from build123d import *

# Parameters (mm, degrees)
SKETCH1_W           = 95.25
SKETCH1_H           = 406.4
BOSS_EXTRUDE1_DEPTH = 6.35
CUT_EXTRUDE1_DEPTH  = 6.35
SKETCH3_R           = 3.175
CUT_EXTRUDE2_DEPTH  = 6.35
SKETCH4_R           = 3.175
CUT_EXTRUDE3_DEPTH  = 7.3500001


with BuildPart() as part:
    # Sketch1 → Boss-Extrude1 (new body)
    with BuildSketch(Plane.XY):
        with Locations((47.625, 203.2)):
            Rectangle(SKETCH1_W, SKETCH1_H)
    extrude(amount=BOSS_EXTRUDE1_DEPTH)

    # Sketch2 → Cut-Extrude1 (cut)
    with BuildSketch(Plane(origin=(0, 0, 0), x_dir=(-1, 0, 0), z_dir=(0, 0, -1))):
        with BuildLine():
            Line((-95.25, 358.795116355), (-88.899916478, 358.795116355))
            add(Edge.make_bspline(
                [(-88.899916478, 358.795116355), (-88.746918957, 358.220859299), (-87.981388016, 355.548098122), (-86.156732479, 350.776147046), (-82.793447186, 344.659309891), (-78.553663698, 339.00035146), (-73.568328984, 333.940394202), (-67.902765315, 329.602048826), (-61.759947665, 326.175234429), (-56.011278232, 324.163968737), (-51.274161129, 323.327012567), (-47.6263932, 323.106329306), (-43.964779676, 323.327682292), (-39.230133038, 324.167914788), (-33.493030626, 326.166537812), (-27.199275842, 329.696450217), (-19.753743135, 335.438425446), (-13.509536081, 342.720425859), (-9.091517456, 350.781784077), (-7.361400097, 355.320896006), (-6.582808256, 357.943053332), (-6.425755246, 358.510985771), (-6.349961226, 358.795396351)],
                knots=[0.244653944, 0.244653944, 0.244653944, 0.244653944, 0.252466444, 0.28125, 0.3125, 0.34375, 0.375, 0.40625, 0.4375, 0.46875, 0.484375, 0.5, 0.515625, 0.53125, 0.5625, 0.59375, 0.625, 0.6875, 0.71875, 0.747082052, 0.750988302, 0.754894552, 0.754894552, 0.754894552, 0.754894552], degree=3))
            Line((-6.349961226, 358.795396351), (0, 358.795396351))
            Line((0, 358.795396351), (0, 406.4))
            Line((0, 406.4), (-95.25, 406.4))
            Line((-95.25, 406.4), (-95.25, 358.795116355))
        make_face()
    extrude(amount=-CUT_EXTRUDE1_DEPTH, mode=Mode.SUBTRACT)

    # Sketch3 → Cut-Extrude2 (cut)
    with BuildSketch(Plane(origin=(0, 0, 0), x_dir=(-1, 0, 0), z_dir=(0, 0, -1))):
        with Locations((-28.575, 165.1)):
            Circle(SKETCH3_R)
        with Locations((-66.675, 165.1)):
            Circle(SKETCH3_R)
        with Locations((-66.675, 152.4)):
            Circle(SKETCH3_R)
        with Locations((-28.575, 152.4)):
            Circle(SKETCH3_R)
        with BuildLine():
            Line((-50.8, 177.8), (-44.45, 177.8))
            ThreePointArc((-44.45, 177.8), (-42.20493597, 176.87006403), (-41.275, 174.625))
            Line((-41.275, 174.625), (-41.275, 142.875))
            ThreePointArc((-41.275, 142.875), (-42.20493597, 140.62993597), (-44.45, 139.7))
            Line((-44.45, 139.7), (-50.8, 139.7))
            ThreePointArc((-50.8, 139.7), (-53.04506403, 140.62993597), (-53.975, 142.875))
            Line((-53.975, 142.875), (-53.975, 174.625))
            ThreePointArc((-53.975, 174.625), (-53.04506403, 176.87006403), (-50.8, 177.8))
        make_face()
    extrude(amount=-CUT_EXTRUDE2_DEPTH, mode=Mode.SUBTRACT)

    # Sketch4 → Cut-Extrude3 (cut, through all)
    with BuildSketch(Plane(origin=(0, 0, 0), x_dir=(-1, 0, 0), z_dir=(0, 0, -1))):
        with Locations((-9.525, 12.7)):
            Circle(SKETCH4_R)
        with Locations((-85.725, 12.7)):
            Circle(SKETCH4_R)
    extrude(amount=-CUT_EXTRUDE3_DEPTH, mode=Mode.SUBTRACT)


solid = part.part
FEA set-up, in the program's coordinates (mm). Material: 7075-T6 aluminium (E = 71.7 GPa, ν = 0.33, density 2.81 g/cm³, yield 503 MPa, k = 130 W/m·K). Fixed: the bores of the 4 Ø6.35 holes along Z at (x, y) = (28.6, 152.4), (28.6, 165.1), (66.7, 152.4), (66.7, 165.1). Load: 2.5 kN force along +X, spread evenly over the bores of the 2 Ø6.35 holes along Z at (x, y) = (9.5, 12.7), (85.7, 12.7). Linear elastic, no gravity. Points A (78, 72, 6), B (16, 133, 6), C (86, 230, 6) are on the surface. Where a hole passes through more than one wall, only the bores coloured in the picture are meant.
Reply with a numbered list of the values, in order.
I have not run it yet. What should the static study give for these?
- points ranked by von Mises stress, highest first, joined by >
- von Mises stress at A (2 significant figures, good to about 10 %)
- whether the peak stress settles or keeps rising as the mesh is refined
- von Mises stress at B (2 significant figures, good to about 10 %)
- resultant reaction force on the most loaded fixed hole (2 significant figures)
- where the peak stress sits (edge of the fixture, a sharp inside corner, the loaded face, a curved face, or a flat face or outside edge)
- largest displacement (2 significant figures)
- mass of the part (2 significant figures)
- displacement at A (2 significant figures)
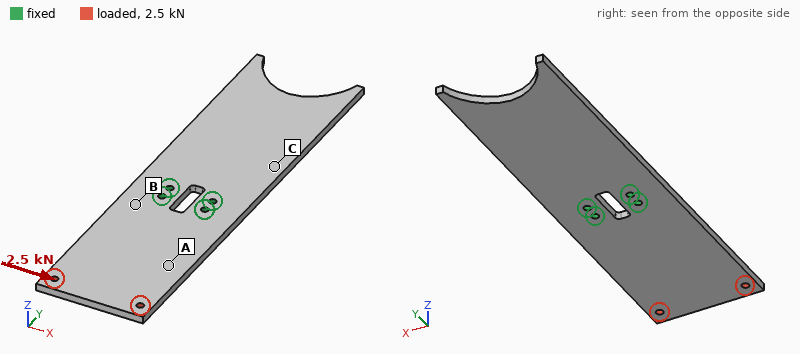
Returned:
1. B > A > C
2. 12 MPa
3. keeps rising
4. 20 MPa
5. 5.3 kN
6. edge of the fixture
7. 0.17 mm
8. 560 g
9. 0.080 mm
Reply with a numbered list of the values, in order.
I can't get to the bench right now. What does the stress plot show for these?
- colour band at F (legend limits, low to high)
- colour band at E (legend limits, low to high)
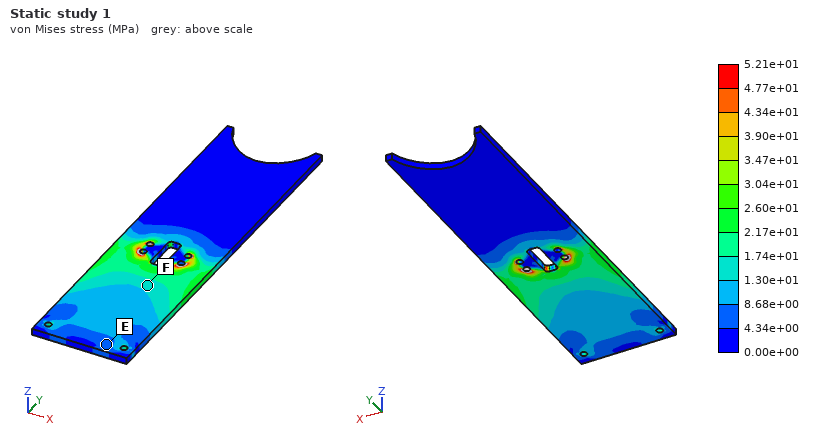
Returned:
1. 1.30e+01 to 1.74e+01 MPa
2. 4.34e+00 to 8.68e+00 MPa
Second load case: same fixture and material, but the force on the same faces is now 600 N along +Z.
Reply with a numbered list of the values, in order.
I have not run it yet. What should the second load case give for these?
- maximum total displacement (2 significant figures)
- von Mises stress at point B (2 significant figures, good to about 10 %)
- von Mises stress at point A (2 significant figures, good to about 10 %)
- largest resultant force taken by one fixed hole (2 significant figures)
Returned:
1. 4.4 mm
2. 110 MPa
3. 54 MPa
4. 1.4 kN
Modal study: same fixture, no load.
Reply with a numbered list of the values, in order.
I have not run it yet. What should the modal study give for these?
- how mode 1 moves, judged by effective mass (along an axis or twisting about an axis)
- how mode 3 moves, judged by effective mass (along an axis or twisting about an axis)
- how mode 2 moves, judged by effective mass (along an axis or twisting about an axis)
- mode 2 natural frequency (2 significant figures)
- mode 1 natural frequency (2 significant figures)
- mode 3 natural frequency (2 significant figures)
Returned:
1. along Z
2. twisting about Y
3. along Z
4. 220 Hz
5. 170 Hz
6. 600 Hz
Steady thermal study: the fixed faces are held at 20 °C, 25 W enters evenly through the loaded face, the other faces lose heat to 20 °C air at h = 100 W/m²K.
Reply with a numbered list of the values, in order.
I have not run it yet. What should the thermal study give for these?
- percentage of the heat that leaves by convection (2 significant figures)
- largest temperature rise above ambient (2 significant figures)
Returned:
1. 86 %
2. 21 K
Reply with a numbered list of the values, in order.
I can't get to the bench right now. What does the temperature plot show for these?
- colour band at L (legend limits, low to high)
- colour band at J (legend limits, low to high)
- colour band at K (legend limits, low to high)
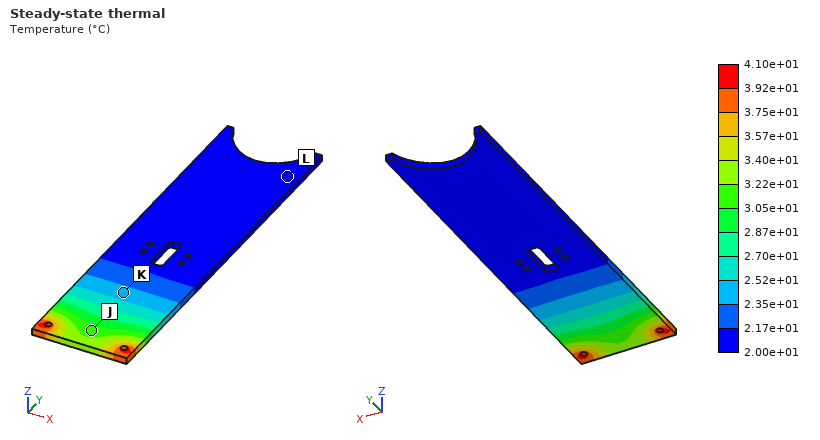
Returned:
1. 2.00e+01 to 2.17e+01 °C
2. 3.05e+01 to 3.22e+01 °C
3. 2.35e+01 to 2.52e+01 °C
